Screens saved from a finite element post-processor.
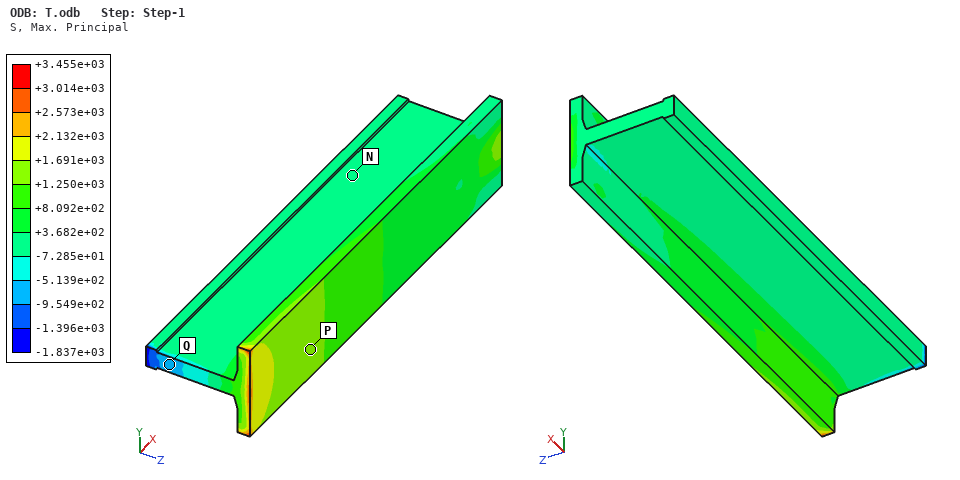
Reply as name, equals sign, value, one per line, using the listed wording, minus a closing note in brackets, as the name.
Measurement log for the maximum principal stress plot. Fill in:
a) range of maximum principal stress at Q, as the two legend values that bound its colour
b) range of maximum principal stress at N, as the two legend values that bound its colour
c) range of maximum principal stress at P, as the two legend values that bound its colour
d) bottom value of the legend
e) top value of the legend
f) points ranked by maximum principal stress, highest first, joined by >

range of maximum principal stress at Q, as the two legend values that bound its colour = -9.549e+02 to -5.139e+02
range of maximum principal stress at N, as the two legend values that bound its colour = -7.285e+01 to +3.682e+02
range of maximum principal stress at P, as the two legend values that bound its colour = +1.250e+03 to +1.691e+03
bottom value of the legend = -1.837e+03
top value of the legend = +3.455e+03
points ranked by maximum principal stress, highest first, joined by > = P > N > Q
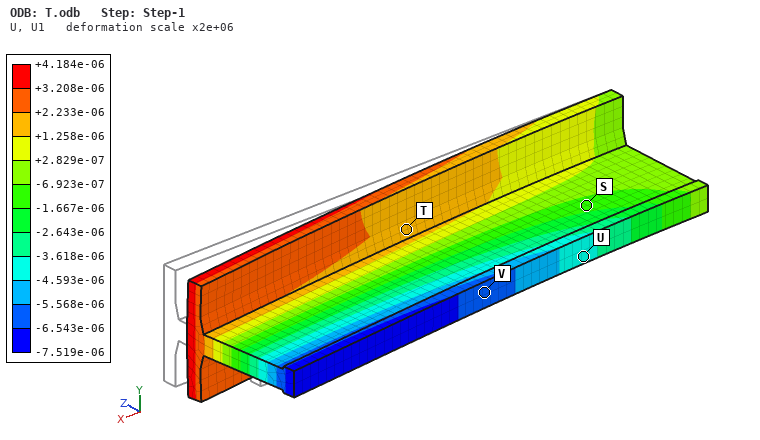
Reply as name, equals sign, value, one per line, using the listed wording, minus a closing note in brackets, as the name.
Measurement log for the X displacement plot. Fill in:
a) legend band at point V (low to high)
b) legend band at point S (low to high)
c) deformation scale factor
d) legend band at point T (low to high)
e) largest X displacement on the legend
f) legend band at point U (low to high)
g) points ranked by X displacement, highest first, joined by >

legend band at point V = -6.543e-06 to -5.568e-06
legend band at point S = -1.667e-06 to -6.923e-07
deformation scale factor = 2e+06
legend band at point T = +1.258e-06 to +2.233e-06
largest X displacement on the legend = +4.184e-06
legend band at point U = -4.593e-06 to -3.618e-06
points ranked by X displacement, highest first, joined by > = T > S > U > V
